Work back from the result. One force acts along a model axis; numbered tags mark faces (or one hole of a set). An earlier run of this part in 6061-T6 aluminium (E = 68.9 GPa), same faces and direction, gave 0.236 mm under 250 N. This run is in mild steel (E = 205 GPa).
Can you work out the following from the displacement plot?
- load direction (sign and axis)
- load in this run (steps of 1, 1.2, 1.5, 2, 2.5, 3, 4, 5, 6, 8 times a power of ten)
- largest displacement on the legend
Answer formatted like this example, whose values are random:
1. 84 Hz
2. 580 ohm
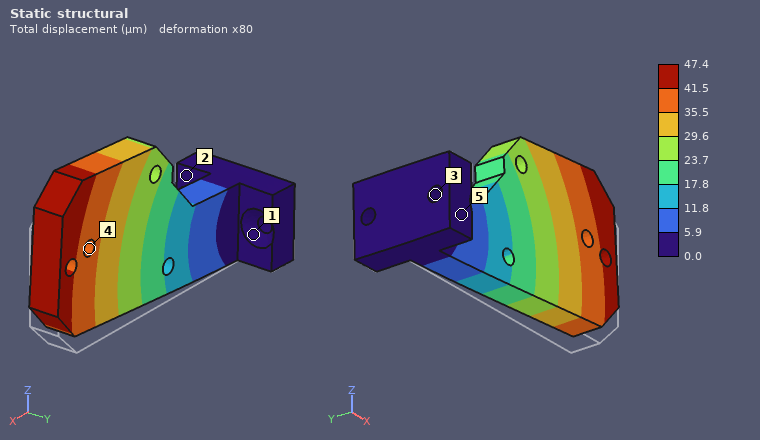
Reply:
1. +Z
2. 150 N
3. 47.4 µm
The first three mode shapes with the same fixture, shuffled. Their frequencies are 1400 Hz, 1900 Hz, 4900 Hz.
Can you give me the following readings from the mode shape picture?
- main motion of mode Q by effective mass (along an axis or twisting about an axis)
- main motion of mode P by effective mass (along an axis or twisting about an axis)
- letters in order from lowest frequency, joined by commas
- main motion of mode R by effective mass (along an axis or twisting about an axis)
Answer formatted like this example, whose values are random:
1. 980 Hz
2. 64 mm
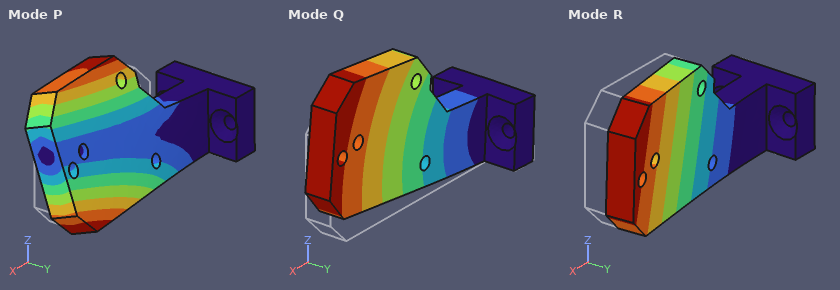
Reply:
1. along Z
2. twisting about X
3. R, Q, P
4. along Y
